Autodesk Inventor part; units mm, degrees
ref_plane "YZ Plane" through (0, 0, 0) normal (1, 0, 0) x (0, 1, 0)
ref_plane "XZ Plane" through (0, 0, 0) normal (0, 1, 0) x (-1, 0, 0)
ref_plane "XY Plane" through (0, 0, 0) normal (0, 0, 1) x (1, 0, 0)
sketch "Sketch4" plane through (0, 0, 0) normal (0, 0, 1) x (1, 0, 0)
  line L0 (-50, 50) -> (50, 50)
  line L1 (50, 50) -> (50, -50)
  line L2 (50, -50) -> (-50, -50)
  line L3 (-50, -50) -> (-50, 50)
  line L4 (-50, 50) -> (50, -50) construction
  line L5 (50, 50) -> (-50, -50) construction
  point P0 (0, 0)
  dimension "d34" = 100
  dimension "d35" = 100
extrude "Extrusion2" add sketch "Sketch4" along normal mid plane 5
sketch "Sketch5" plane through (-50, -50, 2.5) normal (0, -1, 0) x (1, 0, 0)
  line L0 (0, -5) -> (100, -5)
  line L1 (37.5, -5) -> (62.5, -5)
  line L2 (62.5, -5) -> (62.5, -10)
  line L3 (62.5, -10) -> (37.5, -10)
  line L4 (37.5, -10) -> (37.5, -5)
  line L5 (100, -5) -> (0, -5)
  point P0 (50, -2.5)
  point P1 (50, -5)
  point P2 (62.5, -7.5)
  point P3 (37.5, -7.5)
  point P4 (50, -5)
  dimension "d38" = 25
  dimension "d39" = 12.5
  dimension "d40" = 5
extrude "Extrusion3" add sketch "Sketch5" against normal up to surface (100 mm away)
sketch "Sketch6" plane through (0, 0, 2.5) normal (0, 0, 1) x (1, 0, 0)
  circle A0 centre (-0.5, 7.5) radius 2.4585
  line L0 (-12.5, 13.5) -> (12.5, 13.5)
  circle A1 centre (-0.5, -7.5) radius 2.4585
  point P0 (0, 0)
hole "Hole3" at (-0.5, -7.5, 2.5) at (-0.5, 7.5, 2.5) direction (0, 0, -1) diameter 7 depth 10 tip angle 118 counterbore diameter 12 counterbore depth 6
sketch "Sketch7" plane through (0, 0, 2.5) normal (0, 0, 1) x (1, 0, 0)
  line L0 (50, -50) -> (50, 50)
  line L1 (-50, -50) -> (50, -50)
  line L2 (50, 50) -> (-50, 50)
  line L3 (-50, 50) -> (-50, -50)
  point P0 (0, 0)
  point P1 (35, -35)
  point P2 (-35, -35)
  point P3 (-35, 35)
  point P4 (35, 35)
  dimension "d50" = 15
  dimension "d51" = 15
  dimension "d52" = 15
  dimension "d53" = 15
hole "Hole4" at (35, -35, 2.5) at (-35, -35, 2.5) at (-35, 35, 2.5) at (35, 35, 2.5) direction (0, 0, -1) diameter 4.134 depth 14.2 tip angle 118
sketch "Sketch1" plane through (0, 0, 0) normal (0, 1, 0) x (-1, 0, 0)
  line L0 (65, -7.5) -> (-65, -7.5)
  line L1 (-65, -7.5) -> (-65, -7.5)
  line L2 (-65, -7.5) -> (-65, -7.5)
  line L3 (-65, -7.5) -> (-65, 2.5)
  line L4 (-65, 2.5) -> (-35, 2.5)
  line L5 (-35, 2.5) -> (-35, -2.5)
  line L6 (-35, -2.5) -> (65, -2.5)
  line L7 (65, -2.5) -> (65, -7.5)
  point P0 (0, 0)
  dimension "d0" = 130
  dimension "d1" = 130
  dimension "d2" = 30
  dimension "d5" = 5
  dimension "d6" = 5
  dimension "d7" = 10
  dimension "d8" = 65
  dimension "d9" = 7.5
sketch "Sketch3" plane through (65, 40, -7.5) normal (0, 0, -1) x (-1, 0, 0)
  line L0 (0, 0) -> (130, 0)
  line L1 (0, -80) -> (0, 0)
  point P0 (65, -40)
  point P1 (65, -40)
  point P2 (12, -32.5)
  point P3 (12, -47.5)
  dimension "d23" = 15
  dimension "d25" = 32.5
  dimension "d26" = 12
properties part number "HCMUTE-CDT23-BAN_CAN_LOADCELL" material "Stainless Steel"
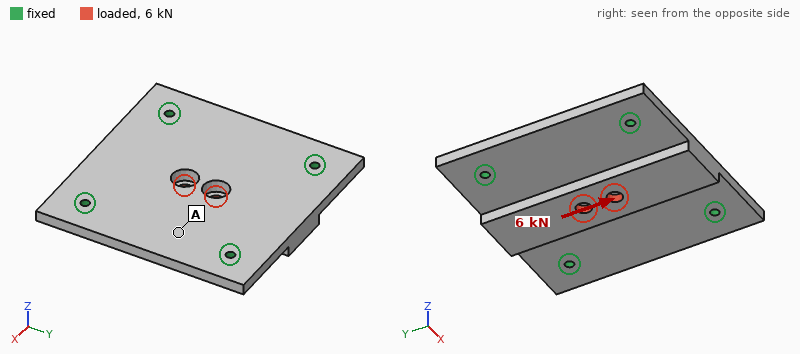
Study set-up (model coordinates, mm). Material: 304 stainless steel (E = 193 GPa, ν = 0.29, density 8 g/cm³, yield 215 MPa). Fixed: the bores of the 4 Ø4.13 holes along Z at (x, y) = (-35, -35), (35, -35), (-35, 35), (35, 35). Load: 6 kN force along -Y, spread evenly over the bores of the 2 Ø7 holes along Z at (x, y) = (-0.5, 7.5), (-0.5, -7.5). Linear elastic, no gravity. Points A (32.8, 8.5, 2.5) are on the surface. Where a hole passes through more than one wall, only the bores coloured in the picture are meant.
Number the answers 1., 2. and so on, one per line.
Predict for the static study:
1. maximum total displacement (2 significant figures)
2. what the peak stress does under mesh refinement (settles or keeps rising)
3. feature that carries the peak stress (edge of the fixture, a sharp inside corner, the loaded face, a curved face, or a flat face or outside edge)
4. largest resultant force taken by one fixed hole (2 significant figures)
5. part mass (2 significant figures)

1. 9.7 µm
2. keeps rising
3. edge of the fixture
4. 1.6 kN
5. 480 g
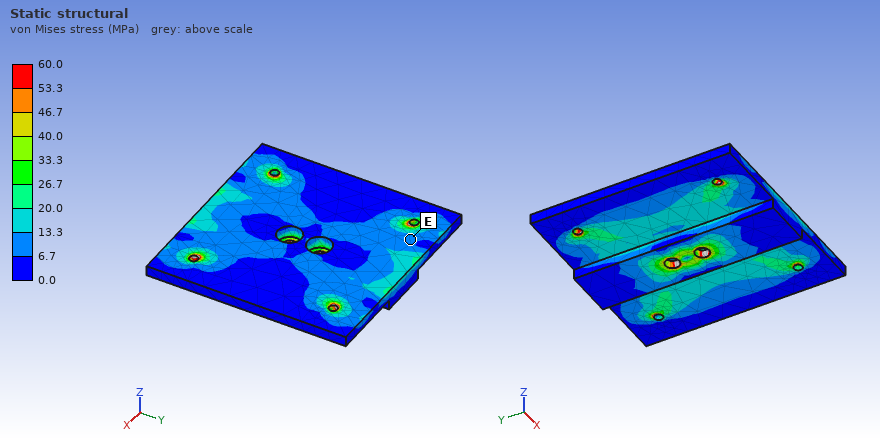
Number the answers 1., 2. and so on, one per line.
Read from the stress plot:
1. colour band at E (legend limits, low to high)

1. 6.7 to 13.3 MPa
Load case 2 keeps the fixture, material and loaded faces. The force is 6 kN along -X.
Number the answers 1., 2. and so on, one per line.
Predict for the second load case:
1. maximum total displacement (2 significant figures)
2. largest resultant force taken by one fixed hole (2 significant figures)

1. 9.1 µm
2. 1.6 kN
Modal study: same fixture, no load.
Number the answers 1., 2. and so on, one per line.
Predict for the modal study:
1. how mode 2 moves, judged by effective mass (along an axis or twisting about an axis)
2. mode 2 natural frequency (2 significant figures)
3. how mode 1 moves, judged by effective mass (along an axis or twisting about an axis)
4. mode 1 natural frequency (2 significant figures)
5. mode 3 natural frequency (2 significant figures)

1. twisting about X
2. 4700 Hz
3. along Z
4. 3600 Hz
5. 5200 Hz
